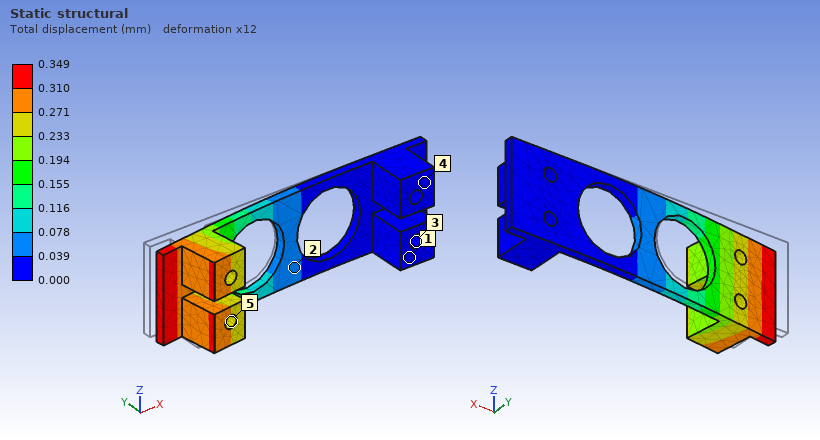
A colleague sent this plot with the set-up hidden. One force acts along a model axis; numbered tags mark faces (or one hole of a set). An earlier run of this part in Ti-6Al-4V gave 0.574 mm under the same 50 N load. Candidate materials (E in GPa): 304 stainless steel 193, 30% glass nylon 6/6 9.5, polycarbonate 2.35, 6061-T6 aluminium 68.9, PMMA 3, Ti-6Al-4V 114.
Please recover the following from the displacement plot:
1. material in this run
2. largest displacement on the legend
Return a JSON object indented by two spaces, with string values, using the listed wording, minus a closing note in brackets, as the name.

{
  "material in this run": "304 stainless steel",
  "largest displacement on the legend": "0.349 mm"
}
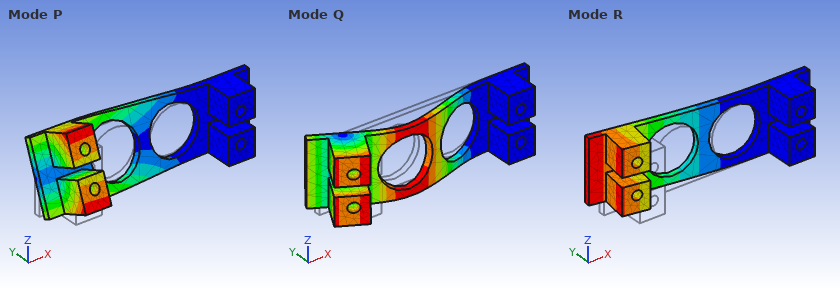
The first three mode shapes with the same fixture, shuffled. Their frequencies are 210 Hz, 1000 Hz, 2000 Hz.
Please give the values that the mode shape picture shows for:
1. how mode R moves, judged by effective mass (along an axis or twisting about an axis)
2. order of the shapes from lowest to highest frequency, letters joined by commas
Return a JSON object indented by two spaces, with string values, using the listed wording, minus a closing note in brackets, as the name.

{
  "how mode R moves, judged by effective mass": "along Y",
  "order of the shapes from lowest to highest frequency, letters joined by commas": "R, P, Q"
}
